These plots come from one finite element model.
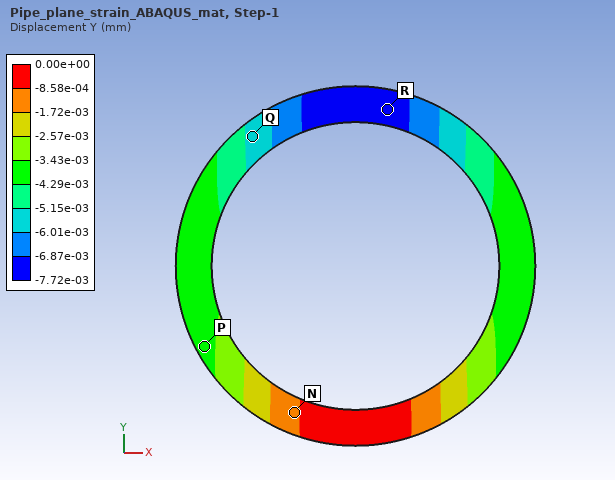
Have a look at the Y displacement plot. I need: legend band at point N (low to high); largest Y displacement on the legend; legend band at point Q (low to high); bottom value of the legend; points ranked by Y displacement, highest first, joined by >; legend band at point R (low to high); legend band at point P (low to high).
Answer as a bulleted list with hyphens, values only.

- -1.72e-03 to -8.58e-04 mm
- 0.00e+00 mm
- -6.01e-03 to -5.15e-03 mm
- -7.72e-03 mm
- N > P > Q > R
- -7.72e-03 to -6.87e-03 mm
- -4.29e-03 to -3.43e-03 mm
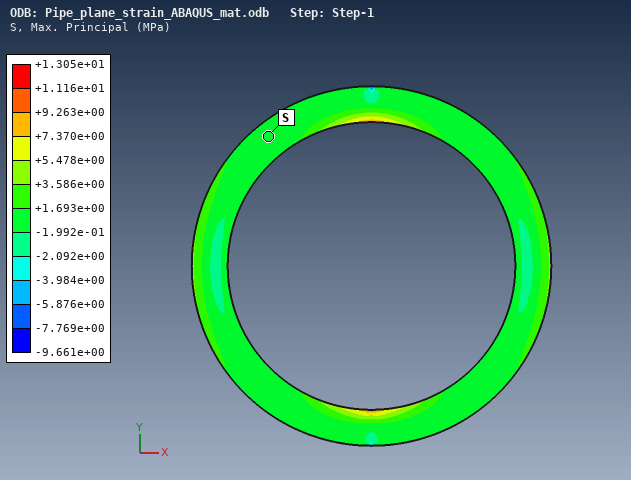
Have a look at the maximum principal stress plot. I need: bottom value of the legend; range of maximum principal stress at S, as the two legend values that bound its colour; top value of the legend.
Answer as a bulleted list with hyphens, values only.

- -9.661e+00 MPa
- -1.992e-01 to +1.693e+00 MPa
- +1.305e+01 MPa
